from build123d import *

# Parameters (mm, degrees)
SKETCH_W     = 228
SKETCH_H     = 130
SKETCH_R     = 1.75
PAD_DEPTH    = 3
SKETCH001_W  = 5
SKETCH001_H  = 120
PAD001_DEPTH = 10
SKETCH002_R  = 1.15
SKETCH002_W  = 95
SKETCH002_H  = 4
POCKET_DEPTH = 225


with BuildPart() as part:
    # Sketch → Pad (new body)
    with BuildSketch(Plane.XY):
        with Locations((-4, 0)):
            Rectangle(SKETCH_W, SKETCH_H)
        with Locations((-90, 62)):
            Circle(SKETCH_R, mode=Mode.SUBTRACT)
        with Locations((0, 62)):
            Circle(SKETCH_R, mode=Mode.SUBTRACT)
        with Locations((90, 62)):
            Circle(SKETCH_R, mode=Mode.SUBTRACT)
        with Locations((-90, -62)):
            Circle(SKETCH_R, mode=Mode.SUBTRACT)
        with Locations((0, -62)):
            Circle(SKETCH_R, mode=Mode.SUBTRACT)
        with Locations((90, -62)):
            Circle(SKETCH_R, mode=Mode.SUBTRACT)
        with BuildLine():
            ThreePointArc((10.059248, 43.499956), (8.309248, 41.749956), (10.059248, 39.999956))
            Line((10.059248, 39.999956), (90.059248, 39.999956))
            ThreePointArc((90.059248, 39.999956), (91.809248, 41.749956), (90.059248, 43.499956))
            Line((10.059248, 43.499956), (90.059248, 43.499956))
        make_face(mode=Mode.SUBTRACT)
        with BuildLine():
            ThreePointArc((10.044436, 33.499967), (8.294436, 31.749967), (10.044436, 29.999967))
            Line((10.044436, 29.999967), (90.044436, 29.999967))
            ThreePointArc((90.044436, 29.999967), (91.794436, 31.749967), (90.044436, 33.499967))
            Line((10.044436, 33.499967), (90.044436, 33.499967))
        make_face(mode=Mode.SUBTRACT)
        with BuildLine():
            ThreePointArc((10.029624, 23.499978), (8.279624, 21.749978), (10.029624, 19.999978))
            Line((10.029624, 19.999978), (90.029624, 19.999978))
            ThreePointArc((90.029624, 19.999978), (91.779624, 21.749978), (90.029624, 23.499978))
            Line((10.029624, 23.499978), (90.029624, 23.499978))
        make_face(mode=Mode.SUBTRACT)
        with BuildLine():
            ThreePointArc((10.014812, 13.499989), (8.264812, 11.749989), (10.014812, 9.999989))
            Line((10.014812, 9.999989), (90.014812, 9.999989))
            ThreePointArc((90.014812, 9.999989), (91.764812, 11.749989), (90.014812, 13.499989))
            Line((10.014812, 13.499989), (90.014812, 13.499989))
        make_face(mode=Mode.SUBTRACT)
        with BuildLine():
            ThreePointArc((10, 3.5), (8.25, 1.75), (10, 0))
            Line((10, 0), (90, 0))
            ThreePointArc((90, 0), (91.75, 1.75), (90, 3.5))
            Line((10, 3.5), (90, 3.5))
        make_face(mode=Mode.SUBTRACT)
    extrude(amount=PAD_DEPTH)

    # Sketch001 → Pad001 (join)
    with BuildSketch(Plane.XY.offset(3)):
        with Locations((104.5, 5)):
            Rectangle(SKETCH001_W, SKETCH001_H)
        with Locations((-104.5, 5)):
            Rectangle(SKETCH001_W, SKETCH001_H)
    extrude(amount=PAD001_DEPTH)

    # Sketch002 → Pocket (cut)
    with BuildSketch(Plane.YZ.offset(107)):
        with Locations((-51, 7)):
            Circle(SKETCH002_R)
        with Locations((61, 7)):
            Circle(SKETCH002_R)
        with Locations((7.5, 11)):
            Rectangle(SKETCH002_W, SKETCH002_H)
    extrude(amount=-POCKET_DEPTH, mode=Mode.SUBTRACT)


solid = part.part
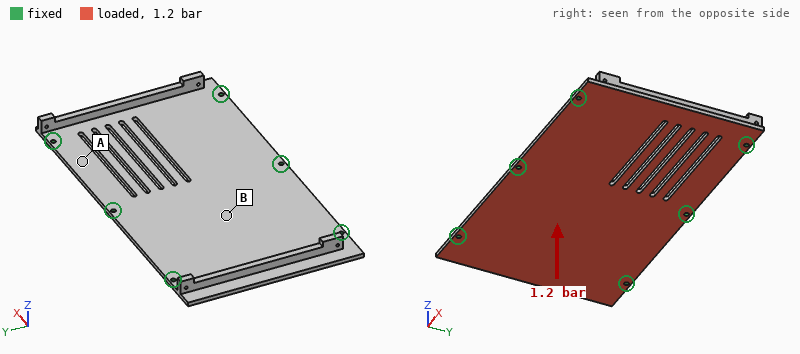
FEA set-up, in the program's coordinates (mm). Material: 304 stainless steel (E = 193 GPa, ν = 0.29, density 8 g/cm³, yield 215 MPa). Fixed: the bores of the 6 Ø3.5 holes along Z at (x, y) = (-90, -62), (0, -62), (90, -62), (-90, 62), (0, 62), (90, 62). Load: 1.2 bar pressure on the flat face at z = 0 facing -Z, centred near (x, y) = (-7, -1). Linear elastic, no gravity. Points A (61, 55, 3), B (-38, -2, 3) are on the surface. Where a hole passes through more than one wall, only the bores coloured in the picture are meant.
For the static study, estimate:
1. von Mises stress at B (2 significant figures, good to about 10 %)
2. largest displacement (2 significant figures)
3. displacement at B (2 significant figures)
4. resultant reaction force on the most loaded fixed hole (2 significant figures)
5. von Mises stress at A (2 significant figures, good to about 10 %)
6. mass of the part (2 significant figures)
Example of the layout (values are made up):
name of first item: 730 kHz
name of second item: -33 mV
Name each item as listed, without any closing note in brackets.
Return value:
von Mises stress at B: 56 MPa
largest displacement: 0.42 mm
displacement at B: 0.30 mm
resultant reaction force on the most loaded fixed hole: 760 N
von Mises stress at A: 20 MPa
mass of the part: 740 g
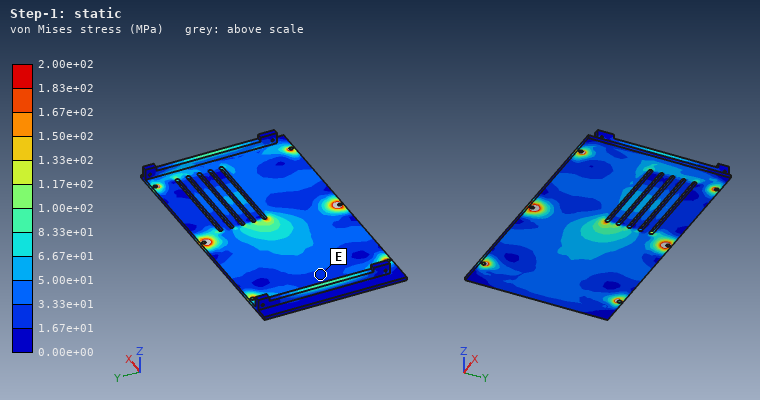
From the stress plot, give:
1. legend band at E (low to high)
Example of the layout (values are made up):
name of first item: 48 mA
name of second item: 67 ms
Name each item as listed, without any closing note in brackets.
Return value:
legend band at E: 1.67e+01 to 3.33e+01 MPa
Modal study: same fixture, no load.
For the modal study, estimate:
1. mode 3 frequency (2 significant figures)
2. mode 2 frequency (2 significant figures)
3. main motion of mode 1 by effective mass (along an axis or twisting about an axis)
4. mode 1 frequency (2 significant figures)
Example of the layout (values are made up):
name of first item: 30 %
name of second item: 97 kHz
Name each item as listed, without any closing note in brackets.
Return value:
mode 3 frequency: 1200 Hz
mode 2 frequency: 950 Hz
main motion of mode 1 by effective mass: along Z
mode 1 frequency: 710 Hz
